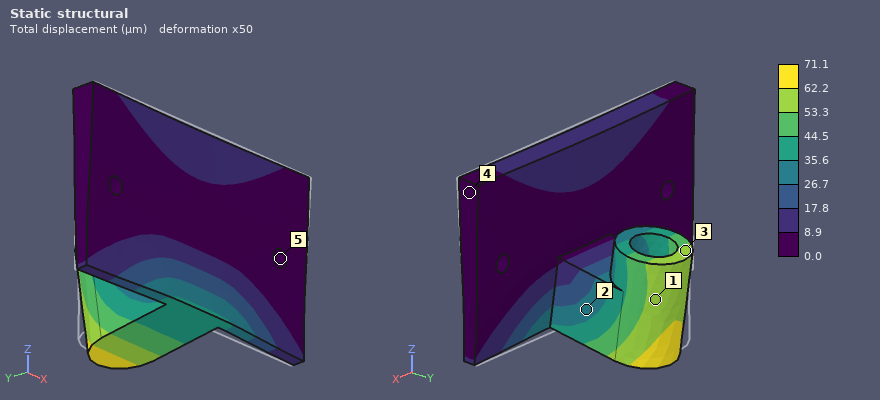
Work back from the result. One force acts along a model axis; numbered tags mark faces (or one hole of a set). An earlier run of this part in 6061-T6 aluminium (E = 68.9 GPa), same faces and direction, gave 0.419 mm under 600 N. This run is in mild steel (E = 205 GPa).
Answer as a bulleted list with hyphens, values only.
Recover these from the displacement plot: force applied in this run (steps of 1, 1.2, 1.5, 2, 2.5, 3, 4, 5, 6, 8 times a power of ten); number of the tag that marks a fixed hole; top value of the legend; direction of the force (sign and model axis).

- 300 N
- 5
- 71.1 µm
- -Z
